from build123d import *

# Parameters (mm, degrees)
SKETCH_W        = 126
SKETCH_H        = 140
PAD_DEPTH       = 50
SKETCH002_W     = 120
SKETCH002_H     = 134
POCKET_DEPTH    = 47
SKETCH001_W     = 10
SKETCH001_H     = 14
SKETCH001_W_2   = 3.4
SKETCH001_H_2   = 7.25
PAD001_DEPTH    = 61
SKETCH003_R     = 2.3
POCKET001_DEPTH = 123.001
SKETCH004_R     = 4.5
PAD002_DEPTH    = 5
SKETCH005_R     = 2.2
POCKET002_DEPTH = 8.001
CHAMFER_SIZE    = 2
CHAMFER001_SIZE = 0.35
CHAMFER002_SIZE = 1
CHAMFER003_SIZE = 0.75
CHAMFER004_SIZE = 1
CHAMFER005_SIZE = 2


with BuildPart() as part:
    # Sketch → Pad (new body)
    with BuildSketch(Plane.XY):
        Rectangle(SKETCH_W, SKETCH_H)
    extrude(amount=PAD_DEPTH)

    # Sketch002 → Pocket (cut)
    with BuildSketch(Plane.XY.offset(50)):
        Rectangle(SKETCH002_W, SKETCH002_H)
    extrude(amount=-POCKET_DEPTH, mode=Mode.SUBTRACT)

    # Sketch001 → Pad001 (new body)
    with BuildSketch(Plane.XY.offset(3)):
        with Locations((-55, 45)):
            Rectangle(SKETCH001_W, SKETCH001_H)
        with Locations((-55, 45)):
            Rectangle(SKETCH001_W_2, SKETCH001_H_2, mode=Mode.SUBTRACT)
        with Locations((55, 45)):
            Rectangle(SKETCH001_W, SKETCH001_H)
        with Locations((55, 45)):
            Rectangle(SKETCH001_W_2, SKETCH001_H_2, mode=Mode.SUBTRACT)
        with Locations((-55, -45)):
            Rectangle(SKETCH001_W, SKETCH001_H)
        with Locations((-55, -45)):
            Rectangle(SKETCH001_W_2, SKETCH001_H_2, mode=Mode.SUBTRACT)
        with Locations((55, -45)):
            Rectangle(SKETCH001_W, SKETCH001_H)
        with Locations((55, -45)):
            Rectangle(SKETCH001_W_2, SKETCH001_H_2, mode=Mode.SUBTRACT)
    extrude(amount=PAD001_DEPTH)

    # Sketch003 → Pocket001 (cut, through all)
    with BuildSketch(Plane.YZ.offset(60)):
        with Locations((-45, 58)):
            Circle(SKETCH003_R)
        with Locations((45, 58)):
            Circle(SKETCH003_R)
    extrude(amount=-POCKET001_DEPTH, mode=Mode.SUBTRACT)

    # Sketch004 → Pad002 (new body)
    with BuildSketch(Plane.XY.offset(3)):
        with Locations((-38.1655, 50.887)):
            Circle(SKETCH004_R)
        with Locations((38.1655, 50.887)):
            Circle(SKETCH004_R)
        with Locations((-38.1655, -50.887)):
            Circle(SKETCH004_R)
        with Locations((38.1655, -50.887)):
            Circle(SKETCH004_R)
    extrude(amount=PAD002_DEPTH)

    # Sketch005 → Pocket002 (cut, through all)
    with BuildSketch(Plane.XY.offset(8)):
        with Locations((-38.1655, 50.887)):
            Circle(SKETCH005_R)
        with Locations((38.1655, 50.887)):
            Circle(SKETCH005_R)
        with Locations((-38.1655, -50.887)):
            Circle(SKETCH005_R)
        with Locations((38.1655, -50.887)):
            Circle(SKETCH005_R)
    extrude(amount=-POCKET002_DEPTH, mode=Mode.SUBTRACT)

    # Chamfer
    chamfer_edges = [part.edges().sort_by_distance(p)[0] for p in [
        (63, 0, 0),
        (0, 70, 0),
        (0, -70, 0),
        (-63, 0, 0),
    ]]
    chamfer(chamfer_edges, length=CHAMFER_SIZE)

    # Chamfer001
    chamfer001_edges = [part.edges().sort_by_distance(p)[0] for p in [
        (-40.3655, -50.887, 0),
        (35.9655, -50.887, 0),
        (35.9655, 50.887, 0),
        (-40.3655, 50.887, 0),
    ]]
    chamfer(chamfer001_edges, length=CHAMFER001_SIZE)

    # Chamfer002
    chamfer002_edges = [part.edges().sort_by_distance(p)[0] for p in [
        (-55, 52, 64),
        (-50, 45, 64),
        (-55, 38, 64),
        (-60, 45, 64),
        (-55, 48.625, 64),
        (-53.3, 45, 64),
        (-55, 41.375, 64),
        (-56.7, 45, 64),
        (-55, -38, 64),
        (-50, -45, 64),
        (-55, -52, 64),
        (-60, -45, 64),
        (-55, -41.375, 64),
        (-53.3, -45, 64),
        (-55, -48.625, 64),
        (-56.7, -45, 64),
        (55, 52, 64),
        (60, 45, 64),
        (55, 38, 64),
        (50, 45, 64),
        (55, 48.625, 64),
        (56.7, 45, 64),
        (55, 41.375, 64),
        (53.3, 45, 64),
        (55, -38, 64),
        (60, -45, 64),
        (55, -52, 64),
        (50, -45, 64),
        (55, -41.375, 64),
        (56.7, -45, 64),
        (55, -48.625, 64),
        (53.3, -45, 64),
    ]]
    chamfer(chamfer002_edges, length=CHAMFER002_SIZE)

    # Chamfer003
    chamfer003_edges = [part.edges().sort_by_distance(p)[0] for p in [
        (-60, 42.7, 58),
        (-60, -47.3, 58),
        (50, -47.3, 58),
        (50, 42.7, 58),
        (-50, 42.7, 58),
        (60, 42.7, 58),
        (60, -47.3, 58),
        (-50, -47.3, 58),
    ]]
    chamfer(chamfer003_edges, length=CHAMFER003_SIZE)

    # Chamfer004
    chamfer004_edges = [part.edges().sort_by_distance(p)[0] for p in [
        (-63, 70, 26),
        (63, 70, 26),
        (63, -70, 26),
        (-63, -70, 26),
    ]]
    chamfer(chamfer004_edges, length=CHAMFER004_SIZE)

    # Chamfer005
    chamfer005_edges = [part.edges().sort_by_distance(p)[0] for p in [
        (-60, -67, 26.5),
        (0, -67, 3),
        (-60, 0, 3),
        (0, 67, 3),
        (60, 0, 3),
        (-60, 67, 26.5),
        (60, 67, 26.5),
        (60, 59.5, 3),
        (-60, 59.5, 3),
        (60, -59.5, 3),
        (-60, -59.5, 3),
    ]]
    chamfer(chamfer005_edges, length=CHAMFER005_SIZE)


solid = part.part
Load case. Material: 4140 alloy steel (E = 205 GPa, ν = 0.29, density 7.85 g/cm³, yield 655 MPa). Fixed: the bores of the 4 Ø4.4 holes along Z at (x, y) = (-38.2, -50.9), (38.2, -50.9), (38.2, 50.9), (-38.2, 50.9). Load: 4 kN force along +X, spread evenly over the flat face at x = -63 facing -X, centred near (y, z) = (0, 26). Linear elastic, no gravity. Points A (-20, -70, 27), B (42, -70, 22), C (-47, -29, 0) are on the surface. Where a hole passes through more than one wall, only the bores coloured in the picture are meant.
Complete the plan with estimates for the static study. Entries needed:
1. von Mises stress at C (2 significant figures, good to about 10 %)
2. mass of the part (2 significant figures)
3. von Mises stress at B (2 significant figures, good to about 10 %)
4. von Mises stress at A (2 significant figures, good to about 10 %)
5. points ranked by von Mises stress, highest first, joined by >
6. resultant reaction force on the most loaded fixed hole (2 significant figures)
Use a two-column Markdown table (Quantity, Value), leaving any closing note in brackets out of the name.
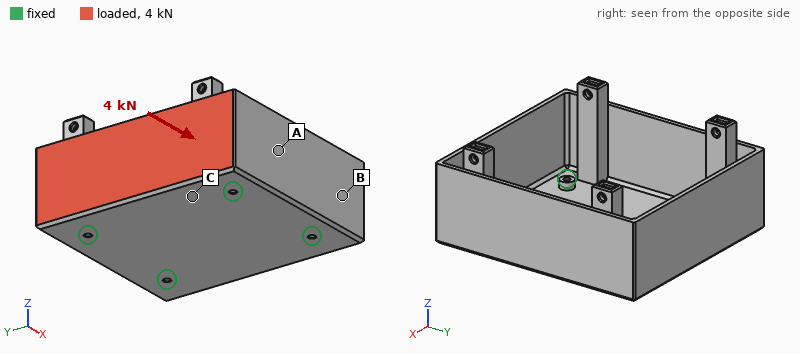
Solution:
| Quantity | Value |
|---|---|
| von Mises stress at C | 32 MPa |
| mass of the part | 1.2 kg |
| von Mises stress at B | 9.3 MPa |
| von Mises stress at A | 22 MPa |
| points ranked by von Mises stress, highest first, joined by > | C > A > B |
| resultant reaction force on the most loaded fixed hole | 1.3 kN |
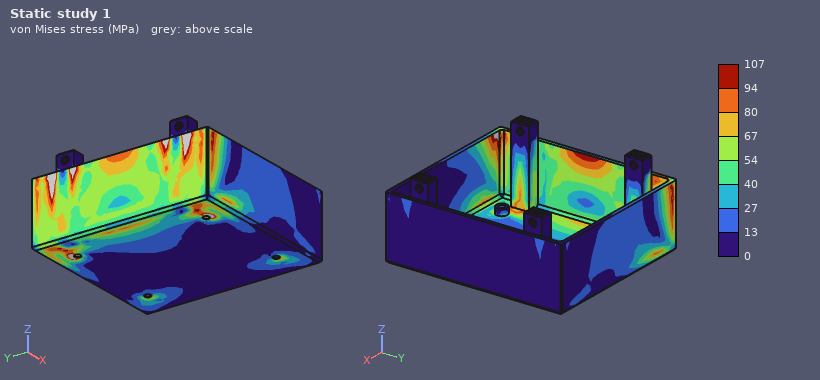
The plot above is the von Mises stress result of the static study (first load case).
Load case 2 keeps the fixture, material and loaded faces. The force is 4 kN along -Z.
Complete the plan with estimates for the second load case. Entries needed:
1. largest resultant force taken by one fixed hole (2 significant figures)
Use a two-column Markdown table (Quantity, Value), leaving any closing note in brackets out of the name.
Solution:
| Quantity | Value |
|---|---|
| largest resultant force taken by one fixed hole | 2.5 kN |
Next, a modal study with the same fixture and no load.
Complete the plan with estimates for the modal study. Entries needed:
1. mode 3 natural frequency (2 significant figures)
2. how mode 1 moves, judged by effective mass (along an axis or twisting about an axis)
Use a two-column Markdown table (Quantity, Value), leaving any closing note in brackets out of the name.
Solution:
| Quantity | Value |
|---|---|
| mode 3 natural frequency | 1500 Hz |
| how mode 1 moves, judged by effective mass | along X |
